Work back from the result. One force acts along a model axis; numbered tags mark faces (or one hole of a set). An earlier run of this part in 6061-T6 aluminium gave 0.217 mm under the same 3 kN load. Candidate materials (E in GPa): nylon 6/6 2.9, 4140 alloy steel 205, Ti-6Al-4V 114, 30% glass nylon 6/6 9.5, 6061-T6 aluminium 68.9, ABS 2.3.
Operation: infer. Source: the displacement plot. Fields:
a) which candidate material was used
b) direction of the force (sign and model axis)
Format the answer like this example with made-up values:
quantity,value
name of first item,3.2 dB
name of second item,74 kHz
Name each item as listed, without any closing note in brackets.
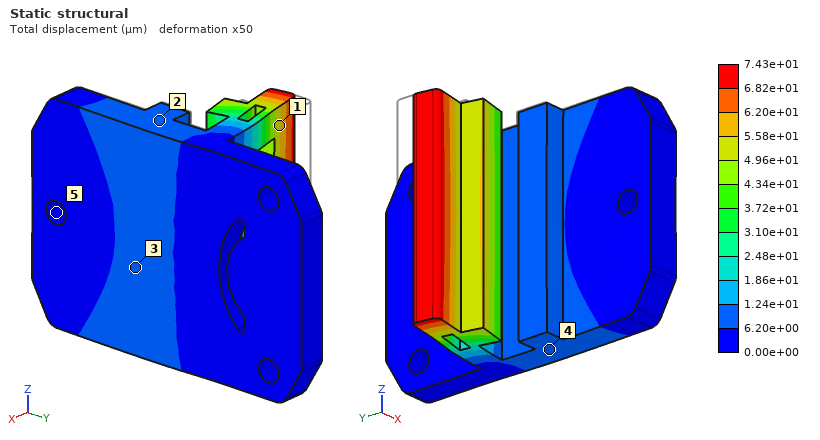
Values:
quantity,value
which candidate material was used,4140 alloy steel
direction of the force,-Y
